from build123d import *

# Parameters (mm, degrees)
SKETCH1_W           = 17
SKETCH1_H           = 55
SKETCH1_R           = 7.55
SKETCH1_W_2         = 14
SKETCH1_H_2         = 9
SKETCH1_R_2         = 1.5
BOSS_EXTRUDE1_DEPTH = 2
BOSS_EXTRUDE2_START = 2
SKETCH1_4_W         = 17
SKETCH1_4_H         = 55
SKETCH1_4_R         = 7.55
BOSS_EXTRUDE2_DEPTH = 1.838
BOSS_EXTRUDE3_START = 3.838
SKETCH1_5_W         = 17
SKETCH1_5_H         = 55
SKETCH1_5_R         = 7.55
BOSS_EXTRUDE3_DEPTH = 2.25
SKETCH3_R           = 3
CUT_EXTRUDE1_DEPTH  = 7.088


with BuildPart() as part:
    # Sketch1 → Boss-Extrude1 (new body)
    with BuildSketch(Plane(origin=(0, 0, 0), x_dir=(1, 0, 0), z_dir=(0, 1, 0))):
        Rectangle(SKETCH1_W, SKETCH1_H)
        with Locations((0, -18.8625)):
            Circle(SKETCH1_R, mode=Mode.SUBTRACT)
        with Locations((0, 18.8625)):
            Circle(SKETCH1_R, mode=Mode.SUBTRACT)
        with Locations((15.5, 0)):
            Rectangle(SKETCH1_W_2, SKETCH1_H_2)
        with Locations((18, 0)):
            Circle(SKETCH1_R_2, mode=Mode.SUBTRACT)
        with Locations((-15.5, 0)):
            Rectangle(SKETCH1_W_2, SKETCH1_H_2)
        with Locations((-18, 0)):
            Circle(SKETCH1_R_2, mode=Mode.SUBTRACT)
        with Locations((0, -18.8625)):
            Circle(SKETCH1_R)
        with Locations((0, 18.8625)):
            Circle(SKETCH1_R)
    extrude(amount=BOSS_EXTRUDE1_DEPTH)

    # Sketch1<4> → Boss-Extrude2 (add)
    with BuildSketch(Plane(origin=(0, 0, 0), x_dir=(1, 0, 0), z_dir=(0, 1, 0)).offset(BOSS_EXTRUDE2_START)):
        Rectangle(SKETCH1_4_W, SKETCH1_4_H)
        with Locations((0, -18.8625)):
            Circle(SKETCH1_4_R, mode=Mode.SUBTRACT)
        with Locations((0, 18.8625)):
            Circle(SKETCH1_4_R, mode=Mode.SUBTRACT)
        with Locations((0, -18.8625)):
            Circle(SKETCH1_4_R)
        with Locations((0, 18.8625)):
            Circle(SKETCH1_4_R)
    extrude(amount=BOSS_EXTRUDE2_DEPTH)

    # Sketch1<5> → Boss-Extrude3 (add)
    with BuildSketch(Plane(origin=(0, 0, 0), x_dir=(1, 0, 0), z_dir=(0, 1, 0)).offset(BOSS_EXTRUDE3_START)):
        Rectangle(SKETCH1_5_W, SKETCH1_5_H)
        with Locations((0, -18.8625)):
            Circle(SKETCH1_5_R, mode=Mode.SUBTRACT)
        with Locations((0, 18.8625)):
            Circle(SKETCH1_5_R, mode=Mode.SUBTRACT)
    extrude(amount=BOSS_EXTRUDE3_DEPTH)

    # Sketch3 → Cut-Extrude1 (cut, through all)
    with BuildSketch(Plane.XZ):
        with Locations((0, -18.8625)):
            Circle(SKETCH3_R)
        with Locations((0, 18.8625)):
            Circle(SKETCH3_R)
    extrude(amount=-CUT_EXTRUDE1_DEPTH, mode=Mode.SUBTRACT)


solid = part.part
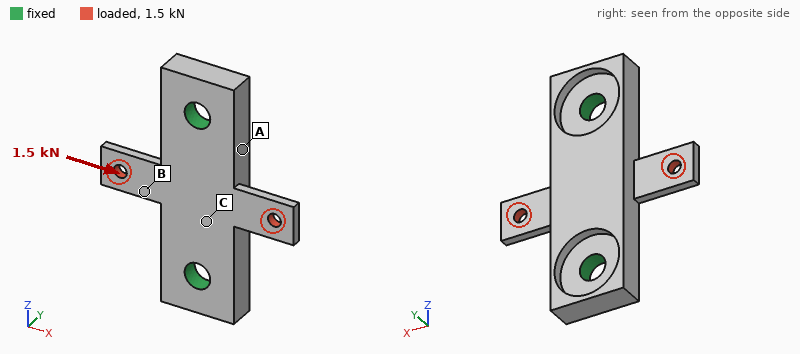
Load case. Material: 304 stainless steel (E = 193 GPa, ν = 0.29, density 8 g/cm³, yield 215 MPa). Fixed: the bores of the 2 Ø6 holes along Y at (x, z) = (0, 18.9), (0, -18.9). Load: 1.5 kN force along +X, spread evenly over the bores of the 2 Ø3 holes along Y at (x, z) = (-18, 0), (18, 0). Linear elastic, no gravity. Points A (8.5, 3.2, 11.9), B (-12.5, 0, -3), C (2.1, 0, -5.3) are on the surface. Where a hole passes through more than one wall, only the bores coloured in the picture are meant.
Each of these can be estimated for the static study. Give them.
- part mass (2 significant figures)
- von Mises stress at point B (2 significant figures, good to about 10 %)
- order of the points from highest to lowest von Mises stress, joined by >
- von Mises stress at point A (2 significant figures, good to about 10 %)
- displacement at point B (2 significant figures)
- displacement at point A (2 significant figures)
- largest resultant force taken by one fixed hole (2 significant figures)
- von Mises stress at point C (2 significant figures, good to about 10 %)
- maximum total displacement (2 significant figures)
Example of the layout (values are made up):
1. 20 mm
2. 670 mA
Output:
1. 41 g
2. 42 MPa
3. B > C > A
4. 10 MPa
5. 7.0 µm
6. 1.9 µm
7. 750 N
8. 25 MPa
9. 12 µm
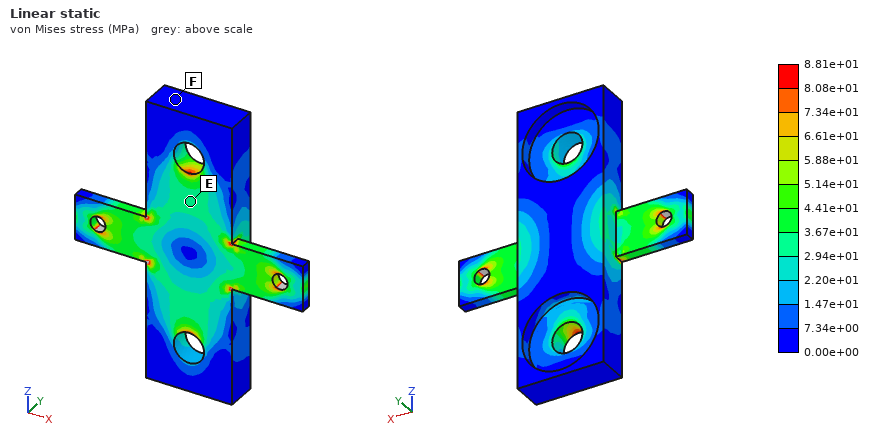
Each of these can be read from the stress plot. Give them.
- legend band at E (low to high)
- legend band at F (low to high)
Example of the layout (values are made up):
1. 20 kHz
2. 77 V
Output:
1. 2.94e+01 to 3.67e+01 MPa
2. 0.00e+00 to 7.34e+00 MPa
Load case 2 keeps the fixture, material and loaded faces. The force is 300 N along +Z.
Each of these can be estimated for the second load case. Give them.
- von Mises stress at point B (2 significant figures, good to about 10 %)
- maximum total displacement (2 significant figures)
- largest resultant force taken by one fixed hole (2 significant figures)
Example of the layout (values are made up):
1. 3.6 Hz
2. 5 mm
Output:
1. 22 MPa
2. 7.5 µm
3. 150 N
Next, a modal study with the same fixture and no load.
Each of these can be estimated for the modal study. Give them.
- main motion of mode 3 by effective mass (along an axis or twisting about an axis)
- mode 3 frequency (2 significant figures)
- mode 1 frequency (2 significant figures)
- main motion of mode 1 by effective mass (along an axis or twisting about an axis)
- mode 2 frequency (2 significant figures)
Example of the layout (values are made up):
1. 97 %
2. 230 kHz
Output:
1. along Y
2. 16 kHz
3. 6500 Hz
4. twisting about Z
5. 7000 Hz
